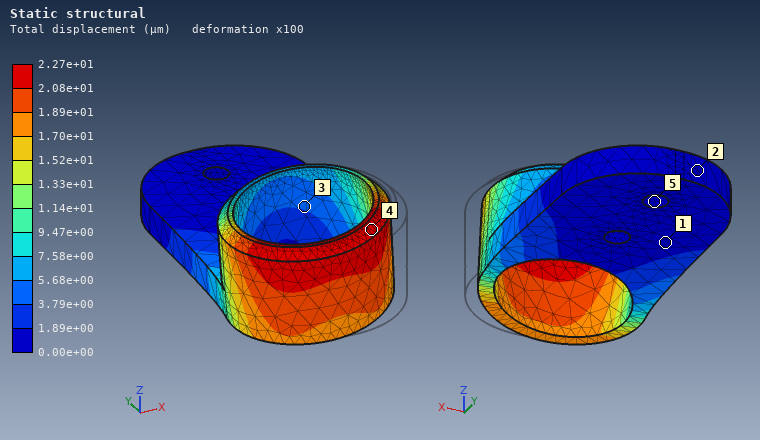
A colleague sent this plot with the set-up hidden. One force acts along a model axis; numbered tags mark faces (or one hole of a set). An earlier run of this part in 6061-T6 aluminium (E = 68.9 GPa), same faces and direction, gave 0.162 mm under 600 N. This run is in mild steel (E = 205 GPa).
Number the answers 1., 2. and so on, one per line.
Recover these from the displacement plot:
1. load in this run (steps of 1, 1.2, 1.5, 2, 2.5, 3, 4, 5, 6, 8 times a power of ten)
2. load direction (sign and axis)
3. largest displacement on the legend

1. 250 N
2. -X
3. 2.27e+01 µm
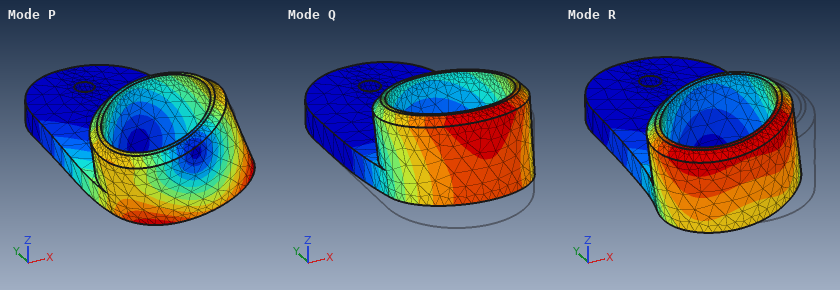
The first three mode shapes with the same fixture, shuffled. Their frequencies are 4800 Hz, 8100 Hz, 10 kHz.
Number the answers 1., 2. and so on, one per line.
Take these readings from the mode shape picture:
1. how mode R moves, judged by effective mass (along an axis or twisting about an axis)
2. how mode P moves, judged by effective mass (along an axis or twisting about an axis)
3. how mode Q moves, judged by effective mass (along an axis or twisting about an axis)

1. along X
2. twisting about Y
3. along Z
